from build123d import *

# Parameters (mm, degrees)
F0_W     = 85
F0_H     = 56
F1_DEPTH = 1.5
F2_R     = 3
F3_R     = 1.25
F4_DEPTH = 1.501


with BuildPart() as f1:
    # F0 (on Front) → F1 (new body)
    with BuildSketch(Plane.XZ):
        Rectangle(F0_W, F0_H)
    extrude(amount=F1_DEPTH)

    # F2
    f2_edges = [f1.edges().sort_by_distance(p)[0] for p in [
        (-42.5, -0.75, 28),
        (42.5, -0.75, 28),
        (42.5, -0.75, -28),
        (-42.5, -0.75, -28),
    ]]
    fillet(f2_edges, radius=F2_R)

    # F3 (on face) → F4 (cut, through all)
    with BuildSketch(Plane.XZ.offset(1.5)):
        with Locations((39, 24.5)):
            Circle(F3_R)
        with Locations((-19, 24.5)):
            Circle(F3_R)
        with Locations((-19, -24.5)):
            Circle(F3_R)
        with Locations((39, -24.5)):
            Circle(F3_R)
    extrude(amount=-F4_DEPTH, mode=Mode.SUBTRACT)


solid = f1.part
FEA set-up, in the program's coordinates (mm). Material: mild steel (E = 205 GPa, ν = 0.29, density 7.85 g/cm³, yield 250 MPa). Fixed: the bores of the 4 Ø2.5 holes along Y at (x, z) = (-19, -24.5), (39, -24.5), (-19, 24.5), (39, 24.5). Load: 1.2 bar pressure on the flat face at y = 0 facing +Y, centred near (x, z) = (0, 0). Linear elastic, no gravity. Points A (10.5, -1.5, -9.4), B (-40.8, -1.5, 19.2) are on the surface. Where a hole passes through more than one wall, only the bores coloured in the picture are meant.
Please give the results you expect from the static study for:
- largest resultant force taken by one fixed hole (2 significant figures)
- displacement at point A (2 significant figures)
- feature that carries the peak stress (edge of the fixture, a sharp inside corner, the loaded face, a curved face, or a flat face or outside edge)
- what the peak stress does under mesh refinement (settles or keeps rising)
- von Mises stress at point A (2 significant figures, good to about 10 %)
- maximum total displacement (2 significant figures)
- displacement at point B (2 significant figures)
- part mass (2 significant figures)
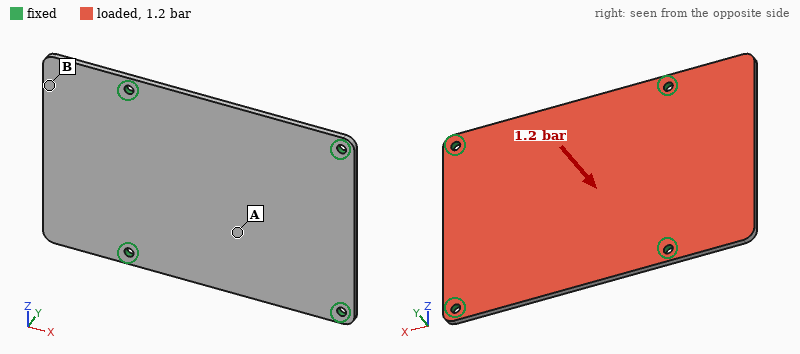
180 N
0.11 mm
edge of the fixture
keeps rising
45 MPa
0.13 mm
0.088 mm
56 g
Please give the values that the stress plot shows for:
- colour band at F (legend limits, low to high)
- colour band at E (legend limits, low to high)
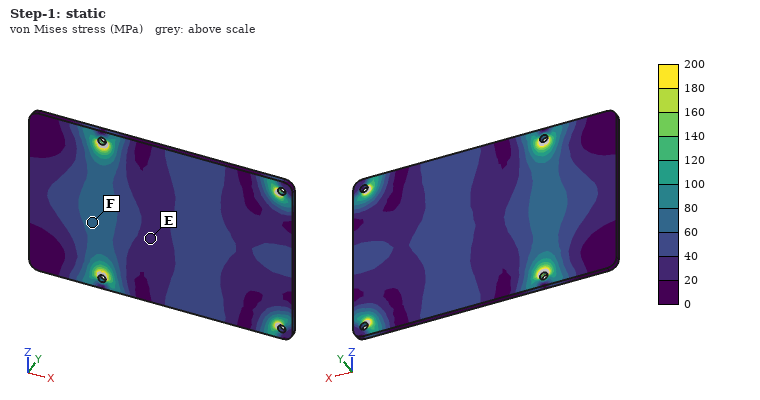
60 to 80 MPa
20 to 40 MPa
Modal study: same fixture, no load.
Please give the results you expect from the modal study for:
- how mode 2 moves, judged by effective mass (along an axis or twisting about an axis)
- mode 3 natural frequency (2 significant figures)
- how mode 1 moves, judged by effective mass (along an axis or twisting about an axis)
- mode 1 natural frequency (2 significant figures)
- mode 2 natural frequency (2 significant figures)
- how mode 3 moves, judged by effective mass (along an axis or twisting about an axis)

along Y
2800 Hz
twisting about Z
1600 Hz
1800 Hz
twisting about X
